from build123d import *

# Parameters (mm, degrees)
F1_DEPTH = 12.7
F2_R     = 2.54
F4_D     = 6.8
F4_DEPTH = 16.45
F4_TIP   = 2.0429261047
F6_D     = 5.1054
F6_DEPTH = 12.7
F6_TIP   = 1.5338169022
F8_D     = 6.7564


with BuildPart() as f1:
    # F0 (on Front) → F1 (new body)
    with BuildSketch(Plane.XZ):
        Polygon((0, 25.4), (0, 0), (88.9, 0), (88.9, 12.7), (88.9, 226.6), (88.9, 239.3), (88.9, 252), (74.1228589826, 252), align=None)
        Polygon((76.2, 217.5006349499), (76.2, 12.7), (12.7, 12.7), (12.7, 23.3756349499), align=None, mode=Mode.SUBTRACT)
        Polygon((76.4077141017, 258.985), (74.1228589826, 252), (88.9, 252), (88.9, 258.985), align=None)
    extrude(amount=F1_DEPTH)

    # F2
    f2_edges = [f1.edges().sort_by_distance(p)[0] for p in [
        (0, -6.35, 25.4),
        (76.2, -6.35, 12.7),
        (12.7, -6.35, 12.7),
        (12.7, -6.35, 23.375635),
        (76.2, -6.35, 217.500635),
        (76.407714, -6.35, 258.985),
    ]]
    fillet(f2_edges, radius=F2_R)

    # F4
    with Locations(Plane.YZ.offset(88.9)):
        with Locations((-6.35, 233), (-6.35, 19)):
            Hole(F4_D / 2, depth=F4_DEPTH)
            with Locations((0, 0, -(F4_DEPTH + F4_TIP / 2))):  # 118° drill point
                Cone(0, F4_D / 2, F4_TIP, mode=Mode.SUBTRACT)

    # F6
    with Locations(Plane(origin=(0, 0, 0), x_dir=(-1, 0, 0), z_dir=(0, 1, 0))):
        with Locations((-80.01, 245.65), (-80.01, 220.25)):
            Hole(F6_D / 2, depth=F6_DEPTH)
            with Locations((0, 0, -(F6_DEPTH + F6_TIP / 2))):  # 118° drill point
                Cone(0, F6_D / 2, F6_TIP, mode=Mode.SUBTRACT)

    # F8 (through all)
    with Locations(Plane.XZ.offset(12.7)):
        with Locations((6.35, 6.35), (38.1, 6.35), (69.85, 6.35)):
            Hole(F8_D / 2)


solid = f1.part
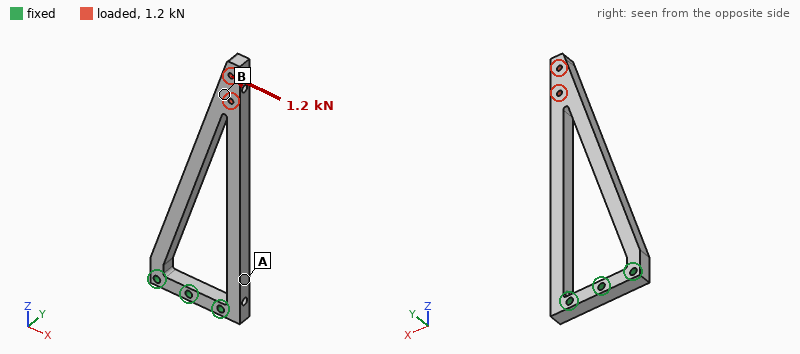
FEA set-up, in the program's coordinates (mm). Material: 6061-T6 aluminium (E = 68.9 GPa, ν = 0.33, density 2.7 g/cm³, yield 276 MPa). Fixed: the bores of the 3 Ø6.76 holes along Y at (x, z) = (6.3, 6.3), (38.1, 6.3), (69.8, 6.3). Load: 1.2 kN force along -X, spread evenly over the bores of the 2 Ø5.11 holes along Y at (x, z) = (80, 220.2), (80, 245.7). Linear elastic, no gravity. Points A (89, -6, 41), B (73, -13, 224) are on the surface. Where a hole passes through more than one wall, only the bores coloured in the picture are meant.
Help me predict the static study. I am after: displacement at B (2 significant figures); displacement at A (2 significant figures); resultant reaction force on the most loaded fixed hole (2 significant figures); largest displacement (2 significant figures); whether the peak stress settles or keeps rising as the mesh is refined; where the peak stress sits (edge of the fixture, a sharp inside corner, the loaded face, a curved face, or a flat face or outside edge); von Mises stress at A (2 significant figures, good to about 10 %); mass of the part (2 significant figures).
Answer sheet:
0.52 mm
0.12 mm
3.5 kN
0.53 mm
keeps rising
edge of the fixture
26 MPa
240 g
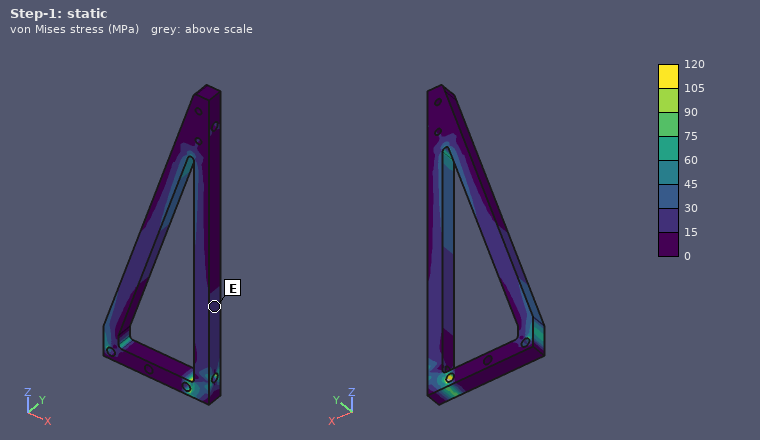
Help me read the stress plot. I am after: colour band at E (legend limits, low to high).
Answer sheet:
15 to 30 MPa
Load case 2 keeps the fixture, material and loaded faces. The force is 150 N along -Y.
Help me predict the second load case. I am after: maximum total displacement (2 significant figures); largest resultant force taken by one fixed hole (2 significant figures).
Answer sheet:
2.5 mm
87 N
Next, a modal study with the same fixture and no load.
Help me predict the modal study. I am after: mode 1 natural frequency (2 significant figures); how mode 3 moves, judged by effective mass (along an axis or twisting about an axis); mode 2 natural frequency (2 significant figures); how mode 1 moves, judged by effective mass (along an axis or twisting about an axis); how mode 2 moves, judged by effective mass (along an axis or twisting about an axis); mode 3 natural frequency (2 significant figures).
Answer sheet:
170 Hz
along Y
580 Hz
along Y
along X
1000 Hz
